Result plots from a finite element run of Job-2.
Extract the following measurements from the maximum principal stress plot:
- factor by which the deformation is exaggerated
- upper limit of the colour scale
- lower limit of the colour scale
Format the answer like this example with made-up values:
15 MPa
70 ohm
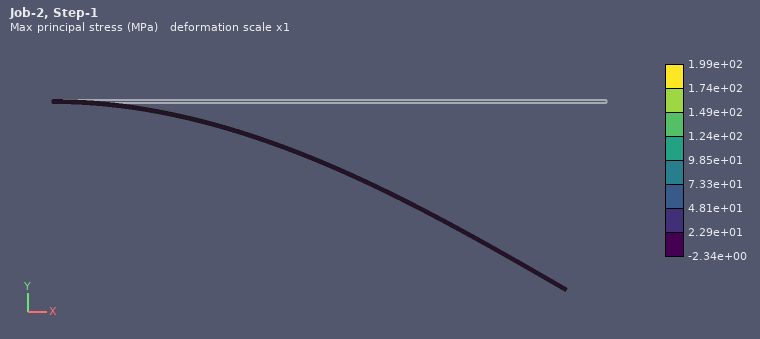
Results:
1
1.99e+02 MPa
-2.34e+00 MPa
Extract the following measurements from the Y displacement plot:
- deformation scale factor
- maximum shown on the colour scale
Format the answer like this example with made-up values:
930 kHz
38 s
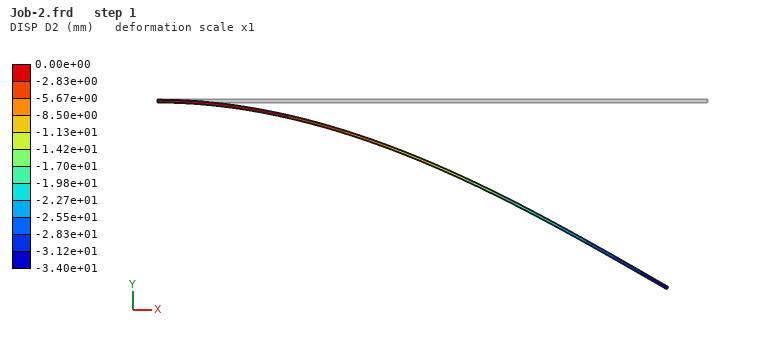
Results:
1
0.00e+00 mm
